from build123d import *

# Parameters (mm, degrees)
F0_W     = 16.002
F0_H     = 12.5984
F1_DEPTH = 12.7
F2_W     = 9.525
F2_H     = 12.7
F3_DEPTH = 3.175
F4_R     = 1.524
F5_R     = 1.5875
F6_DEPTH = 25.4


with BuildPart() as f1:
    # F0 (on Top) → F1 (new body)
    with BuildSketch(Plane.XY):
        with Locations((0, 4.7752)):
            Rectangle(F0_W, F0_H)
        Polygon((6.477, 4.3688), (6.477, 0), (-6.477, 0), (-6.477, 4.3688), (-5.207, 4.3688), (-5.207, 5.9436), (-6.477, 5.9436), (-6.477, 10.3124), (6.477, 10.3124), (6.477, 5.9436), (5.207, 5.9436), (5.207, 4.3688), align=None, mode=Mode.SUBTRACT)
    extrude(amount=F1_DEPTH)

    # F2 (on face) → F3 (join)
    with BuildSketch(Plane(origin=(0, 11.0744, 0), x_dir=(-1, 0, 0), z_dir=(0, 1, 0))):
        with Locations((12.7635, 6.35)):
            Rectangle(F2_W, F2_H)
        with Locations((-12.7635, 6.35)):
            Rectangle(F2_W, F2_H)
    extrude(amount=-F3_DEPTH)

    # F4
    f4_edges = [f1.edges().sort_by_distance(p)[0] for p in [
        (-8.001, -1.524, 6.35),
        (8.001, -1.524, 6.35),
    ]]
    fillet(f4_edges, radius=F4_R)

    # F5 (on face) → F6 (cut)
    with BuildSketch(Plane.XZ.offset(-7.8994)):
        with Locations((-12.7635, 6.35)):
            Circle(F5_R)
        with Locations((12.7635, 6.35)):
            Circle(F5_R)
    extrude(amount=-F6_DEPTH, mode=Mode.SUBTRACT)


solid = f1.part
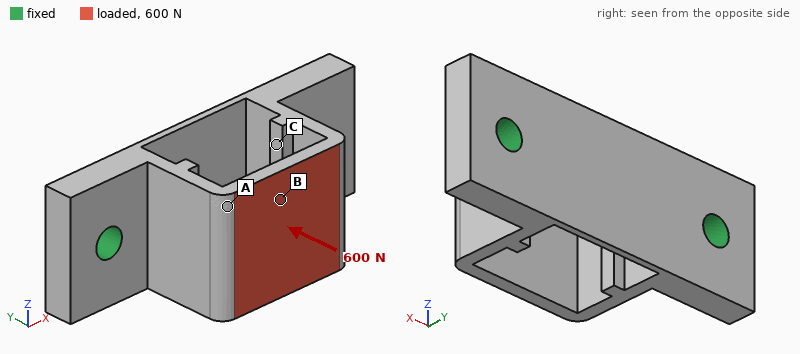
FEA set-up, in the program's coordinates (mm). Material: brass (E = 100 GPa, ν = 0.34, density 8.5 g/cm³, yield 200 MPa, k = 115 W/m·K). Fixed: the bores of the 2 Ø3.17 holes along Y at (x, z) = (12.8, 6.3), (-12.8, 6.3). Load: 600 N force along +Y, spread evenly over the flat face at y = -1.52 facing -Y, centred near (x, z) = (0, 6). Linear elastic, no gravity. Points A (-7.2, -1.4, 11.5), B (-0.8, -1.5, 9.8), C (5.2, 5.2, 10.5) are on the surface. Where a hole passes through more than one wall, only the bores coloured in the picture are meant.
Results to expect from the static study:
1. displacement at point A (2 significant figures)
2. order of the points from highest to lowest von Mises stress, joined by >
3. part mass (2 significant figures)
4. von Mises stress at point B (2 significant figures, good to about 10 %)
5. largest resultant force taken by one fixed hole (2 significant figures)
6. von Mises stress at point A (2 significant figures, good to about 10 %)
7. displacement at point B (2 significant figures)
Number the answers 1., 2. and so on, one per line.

1. 5.2 µm
2. B > A > C
3. 14 g
4. 100 MPa
5. 300 N
6. 44 MPa
7. 28 µm
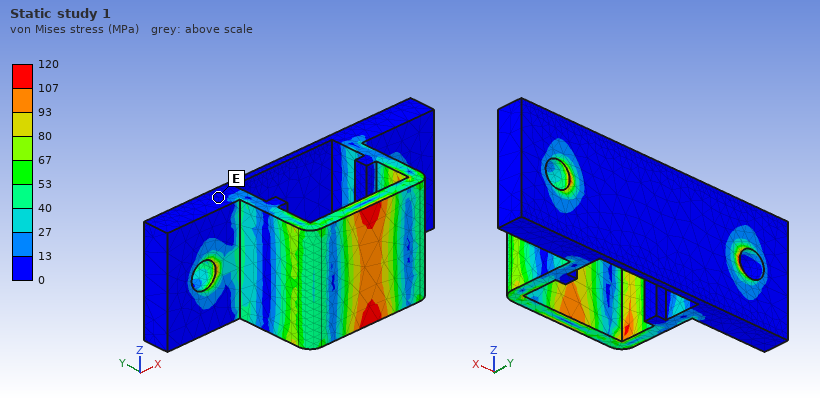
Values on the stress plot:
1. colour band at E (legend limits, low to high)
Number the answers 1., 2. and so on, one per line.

1. 0 to 13 MPa
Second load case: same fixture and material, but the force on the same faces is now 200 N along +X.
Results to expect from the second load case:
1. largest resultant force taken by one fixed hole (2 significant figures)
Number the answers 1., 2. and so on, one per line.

1. 120 N
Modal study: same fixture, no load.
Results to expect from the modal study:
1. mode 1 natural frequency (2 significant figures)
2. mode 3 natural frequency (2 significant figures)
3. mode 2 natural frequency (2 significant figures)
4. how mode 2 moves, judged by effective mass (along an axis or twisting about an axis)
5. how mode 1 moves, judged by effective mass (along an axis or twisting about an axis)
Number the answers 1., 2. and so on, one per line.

1. 7100 Hz
2. 12 kHz
3. 9300 Hz
4. along Z
5. along X
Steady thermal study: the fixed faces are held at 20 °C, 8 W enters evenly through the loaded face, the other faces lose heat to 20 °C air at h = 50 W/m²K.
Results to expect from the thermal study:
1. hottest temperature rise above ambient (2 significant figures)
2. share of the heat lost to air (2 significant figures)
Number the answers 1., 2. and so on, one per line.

1. 26 K
2. 9.3 %
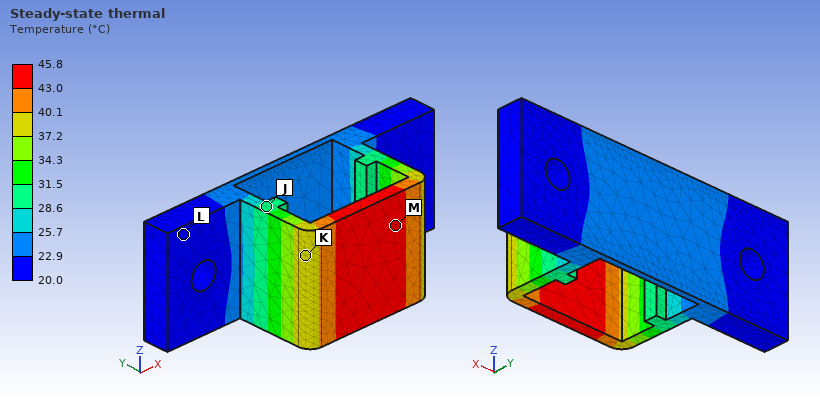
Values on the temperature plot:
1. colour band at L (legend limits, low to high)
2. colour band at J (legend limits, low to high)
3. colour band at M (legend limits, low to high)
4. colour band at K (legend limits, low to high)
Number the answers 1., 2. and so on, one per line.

1. 20.0 to 22.9 °C
2. 28.6 to 31.5 °C
3. 43.0 to 45.8 °C
4. 37.2 to 40.1 °C
